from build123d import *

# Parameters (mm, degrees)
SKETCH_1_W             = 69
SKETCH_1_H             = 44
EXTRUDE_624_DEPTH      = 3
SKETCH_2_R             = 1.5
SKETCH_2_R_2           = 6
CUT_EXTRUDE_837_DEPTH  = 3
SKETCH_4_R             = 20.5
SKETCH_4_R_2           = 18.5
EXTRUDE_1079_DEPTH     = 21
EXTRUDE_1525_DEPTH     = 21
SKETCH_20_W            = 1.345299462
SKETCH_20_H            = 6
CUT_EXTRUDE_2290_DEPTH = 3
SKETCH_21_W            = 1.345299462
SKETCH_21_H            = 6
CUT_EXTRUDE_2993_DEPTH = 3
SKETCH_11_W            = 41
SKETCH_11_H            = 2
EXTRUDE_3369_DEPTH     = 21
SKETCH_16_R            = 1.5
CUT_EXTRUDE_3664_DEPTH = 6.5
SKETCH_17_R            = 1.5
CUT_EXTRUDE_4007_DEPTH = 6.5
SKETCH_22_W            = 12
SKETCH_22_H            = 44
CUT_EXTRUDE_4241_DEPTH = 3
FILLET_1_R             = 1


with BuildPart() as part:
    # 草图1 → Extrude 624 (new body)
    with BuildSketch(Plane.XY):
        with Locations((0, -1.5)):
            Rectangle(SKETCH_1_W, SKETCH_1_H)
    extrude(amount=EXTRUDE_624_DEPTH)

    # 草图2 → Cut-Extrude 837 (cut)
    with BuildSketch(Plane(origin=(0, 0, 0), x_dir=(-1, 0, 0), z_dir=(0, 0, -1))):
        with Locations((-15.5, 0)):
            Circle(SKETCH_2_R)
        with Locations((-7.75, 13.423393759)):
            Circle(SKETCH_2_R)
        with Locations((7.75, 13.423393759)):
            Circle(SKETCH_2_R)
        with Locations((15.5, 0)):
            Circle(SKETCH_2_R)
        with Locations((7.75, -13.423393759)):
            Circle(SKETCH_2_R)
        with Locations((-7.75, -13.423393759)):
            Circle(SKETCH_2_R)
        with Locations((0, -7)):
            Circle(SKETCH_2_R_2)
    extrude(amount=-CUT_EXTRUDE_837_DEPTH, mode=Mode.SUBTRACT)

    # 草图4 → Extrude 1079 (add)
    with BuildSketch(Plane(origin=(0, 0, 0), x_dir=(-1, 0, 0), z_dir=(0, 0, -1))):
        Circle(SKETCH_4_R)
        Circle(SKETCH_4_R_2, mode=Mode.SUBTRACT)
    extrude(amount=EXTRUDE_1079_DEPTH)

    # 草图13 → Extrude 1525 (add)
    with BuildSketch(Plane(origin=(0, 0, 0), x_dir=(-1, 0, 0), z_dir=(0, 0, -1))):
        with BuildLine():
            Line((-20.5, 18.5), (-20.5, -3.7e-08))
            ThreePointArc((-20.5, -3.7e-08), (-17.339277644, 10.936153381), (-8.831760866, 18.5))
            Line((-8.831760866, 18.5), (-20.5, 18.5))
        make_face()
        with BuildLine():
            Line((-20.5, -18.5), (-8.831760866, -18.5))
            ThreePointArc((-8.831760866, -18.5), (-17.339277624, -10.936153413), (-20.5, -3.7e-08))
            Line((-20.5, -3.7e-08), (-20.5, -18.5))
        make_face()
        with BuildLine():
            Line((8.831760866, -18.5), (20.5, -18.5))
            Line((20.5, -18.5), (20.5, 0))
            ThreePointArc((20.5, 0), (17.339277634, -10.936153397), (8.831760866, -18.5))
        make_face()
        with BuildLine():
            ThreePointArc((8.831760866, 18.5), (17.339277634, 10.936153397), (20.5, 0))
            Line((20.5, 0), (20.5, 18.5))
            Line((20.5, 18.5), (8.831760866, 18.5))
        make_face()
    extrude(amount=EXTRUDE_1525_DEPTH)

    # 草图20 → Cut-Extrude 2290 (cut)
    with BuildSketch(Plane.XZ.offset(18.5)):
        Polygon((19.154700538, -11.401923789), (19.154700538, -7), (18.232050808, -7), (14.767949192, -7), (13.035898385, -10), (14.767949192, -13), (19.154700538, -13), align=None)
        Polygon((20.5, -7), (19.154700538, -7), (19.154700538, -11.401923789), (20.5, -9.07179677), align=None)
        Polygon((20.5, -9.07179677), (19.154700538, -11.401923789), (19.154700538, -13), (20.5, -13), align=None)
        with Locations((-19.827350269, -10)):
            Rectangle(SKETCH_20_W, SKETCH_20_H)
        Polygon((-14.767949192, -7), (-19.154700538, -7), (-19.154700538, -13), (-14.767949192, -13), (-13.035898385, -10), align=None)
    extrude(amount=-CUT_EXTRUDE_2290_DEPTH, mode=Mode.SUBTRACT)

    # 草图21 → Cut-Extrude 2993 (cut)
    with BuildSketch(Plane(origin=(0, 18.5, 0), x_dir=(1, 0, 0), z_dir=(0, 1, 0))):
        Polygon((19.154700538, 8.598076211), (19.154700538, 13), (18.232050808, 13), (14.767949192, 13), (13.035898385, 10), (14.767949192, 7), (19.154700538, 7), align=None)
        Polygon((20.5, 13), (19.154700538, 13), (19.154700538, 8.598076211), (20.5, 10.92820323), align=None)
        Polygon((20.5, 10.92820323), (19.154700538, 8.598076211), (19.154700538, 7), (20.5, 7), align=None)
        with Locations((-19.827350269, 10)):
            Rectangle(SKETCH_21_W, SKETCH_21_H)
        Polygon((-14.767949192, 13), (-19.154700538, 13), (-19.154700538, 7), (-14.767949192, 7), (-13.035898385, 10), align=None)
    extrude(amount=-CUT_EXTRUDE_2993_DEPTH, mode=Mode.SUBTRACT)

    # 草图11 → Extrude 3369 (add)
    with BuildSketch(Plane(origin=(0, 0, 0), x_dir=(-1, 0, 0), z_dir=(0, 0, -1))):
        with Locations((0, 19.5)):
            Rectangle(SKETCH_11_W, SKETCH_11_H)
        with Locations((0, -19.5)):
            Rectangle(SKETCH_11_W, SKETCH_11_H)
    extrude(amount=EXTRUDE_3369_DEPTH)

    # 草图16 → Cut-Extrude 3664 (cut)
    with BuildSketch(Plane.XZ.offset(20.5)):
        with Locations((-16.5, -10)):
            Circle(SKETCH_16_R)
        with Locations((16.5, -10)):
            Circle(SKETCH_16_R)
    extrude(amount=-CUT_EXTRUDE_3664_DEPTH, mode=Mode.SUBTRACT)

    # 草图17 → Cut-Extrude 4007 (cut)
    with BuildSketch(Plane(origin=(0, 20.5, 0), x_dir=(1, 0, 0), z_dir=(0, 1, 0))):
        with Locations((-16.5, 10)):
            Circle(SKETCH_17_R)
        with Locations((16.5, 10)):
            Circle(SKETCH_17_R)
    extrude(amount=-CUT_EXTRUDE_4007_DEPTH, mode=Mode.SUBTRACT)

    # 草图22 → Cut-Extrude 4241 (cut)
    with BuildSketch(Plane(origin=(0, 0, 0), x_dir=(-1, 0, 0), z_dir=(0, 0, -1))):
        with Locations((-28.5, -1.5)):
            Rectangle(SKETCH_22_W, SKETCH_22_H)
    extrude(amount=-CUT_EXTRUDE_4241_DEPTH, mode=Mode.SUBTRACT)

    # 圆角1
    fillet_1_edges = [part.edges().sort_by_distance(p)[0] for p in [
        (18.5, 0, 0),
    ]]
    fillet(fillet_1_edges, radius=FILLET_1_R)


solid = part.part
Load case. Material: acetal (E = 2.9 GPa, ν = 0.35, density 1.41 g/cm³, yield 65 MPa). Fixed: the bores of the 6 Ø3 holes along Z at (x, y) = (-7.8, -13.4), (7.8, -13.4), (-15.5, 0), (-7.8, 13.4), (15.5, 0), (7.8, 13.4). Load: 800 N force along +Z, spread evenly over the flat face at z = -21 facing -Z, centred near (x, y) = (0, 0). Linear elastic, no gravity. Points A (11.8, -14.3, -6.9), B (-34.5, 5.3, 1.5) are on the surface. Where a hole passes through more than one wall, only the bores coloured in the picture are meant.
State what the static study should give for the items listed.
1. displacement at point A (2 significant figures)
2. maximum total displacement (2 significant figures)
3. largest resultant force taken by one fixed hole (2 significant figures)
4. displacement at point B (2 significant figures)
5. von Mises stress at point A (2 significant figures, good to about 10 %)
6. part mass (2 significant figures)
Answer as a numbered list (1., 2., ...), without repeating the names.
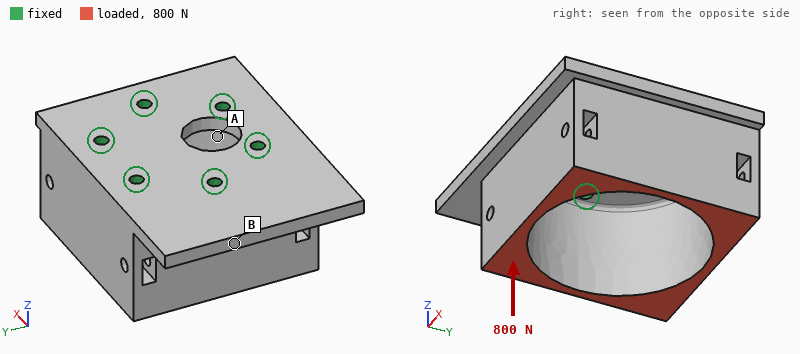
1. 35 µm
2. 68 µm
3. 140 N
4. 65 µm
5. 3.5 MPa
6. 27 g
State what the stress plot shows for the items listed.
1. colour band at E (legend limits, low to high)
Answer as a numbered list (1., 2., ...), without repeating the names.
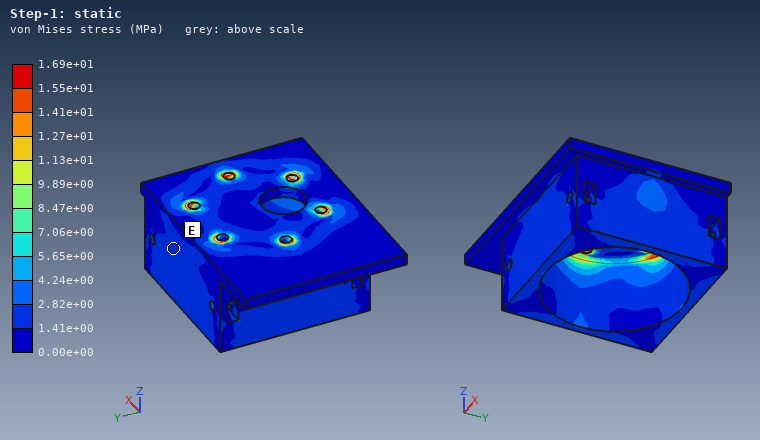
1. 1.41e+00 to 2.82e+00 MPa
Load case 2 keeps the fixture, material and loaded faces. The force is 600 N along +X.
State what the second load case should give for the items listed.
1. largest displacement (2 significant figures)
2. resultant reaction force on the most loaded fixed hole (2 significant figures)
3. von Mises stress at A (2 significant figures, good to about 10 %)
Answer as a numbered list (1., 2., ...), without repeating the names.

1. 0.24 mm
2. 250 N
3. 4.1 MPa
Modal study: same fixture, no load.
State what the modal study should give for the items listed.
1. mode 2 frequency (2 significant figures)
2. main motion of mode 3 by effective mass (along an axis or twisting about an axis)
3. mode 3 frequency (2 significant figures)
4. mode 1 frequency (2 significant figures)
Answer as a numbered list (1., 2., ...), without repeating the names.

1. 2100 Hz
2. along Y
3. 2800 Hz
4. 1900 Hz
